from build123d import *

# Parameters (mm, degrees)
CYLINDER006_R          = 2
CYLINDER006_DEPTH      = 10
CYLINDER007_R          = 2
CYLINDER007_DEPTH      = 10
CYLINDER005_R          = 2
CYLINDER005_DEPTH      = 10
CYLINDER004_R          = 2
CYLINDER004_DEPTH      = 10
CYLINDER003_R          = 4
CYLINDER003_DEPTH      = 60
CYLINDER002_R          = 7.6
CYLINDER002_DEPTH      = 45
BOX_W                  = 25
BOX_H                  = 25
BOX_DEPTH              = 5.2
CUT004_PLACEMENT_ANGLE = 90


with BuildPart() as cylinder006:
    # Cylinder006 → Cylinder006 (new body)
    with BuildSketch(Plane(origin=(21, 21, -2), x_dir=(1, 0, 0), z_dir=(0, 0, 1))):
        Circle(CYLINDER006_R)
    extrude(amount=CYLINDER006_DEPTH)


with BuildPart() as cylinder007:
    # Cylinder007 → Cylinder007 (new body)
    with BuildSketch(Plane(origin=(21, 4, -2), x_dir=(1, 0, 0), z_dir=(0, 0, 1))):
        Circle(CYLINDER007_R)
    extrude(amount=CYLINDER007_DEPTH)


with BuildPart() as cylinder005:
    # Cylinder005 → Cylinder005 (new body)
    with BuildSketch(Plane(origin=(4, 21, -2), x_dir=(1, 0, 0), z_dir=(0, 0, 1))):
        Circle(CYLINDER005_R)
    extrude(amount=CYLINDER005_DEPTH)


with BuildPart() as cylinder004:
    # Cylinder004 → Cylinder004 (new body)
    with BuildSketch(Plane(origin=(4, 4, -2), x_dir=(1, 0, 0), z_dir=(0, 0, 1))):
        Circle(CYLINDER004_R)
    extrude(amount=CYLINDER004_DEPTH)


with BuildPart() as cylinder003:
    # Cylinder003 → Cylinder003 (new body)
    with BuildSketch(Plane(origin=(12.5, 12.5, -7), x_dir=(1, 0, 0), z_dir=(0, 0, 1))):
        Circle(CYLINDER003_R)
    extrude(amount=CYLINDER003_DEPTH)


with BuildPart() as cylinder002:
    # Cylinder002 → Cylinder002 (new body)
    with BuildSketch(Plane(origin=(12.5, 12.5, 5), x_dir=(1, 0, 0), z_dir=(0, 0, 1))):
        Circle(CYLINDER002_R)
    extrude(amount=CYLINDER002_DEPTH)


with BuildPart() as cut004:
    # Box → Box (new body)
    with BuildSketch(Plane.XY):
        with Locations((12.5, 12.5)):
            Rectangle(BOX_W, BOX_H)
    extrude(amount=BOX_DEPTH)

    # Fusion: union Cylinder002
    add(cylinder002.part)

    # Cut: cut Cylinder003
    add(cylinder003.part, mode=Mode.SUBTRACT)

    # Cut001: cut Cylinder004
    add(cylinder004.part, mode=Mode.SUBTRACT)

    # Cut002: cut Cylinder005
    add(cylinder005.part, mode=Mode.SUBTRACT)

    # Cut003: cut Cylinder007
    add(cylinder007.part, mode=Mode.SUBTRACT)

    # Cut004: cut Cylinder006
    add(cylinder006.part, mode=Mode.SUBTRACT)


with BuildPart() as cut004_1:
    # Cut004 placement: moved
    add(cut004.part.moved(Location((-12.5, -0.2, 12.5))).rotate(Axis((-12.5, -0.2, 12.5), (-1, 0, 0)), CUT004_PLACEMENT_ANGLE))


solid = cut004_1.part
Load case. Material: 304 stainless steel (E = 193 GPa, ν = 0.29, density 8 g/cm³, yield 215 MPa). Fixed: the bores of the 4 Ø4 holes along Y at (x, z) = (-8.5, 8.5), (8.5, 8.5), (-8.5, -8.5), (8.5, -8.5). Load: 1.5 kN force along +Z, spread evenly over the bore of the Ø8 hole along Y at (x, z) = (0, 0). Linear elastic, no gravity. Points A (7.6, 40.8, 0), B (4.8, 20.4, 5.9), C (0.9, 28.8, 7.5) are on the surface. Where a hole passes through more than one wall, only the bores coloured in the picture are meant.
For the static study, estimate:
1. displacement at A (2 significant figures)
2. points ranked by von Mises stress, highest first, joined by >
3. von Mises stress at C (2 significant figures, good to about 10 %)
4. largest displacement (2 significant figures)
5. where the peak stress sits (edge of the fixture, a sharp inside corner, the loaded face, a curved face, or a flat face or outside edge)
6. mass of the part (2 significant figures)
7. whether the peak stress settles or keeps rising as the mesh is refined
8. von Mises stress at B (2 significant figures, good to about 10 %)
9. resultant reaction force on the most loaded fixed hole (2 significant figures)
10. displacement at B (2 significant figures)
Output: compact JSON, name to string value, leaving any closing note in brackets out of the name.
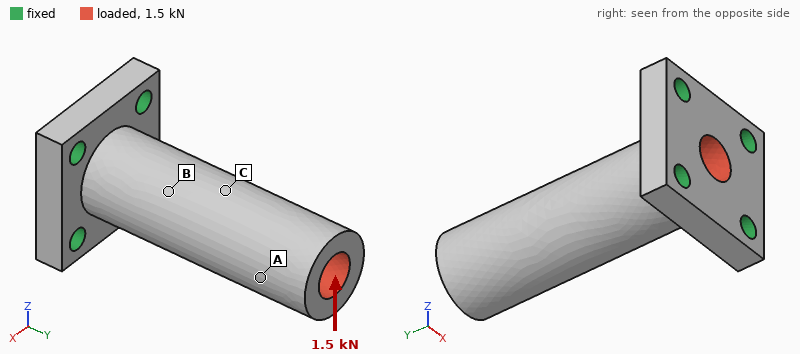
{"displacement at A": "44 µm", "points ranked by von Mises stress, highest first, joined by >": "B > C > A", "von Mises stress at C": "20 MPa", "largest displacement": "58 µm", "where the peak stress sits": "edge of the fixture", "mass of the part": "69 g", "whether the peak stress settles or keeps rising as the mesh is refined": "keeps rising", "von Mises stress at B": "33 MPa", "resultant reaction force on the most loaded fixed hole": "1.2 kN", "displacement at B": "17 µm"}
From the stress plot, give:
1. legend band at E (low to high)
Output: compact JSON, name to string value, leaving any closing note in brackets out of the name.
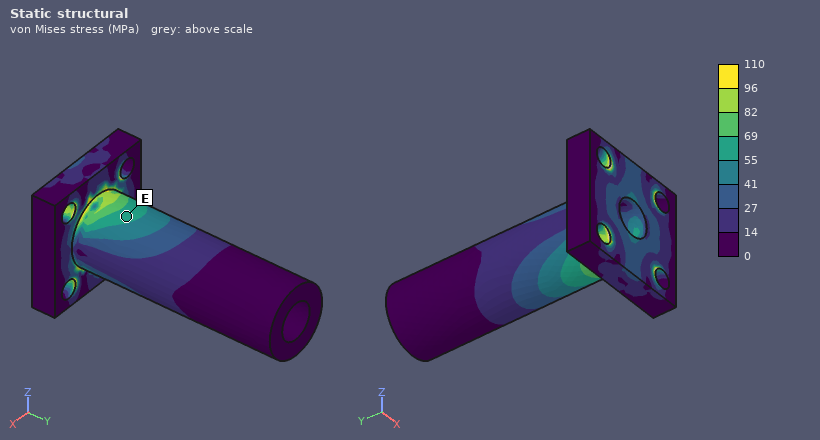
{"legend band at E": "55 to 69 MPa"}
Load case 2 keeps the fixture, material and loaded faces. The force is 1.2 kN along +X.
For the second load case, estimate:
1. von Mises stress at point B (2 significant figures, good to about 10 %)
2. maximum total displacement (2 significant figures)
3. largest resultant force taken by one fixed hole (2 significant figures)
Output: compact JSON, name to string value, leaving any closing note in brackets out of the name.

{"von Mises stress at point B": "23 MPa", "maximum total displacement": "46 µm", "largest resultant force taken by one fixed hole": "970 N"}
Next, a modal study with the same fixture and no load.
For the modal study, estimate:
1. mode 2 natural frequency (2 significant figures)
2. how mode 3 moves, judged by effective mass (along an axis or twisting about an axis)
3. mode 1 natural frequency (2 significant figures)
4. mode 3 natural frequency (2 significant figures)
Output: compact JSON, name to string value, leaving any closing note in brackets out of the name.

{"mode 2 natural frequency": "4300 Hz", "how mode 3 moves, judged by effective mass": "twisting about Y", "mode 1 natural frequency": "4300 Hz", "mode 3 natural frequency": "16 kHz"}
